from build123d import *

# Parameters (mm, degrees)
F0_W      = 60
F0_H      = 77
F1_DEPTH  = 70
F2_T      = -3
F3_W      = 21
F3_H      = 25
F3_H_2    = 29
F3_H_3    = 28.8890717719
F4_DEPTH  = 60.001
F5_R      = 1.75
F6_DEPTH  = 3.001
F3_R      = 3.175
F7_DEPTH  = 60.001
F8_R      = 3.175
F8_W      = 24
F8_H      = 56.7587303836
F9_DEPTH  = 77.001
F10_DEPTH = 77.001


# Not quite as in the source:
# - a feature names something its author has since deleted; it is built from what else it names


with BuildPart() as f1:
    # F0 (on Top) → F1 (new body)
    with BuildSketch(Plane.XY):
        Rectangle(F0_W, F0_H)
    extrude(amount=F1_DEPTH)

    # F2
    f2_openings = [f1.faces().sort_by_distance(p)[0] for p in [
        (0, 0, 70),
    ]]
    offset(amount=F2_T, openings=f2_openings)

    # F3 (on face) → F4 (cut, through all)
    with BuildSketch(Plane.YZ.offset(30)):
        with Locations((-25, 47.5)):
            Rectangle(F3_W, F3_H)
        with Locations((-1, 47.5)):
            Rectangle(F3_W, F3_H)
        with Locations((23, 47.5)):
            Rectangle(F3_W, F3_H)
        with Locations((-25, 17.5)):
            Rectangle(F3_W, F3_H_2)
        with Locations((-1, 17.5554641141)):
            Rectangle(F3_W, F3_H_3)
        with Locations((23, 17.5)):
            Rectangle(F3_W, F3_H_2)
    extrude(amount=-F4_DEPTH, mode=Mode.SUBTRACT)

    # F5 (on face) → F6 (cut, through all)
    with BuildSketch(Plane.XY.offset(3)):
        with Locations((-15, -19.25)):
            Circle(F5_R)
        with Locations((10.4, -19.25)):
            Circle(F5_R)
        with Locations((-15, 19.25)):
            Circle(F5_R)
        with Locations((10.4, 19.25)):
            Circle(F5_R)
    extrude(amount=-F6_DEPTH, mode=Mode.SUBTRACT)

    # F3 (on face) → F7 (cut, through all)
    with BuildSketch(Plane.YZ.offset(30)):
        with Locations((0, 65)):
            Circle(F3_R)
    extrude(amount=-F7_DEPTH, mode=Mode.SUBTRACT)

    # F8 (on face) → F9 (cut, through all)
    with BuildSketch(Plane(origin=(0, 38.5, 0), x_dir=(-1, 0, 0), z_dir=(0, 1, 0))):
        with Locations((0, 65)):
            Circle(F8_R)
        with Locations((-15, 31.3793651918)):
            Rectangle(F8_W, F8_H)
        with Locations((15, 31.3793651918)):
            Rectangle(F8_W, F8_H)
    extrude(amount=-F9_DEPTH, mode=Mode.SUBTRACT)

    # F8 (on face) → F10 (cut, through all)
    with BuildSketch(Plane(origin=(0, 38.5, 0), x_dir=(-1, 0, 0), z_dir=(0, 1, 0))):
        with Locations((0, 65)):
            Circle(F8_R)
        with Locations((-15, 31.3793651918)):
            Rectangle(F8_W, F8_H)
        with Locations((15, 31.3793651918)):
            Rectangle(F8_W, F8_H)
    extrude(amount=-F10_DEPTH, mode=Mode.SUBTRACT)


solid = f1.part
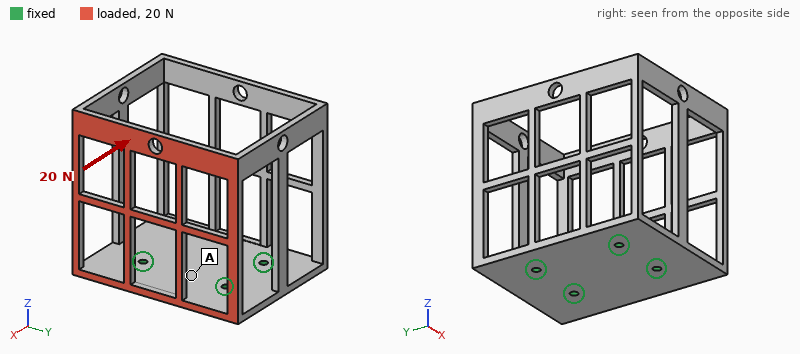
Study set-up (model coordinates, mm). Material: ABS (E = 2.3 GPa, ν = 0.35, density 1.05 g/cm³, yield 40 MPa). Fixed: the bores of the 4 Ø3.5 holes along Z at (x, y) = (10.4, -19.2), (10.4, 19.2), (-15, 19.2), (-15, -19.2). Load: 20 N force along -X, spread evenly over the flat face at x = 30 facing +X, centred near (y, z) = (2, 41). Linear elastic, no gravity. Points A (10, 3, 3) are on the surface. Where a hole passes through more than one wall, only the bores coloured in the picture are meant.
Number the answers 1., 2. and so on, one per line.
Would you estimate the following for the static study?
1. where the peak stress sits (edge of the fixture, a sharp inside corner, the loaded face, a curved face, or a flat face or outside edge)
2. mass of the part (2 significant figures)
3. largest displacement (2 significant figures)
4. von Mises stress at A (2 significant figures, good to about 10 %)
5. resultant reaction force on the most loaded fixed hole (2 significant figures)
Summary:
1. the loaded face
2. 31 g
3. 1.4 mm
4. 0.91 MPa
5. 13 N
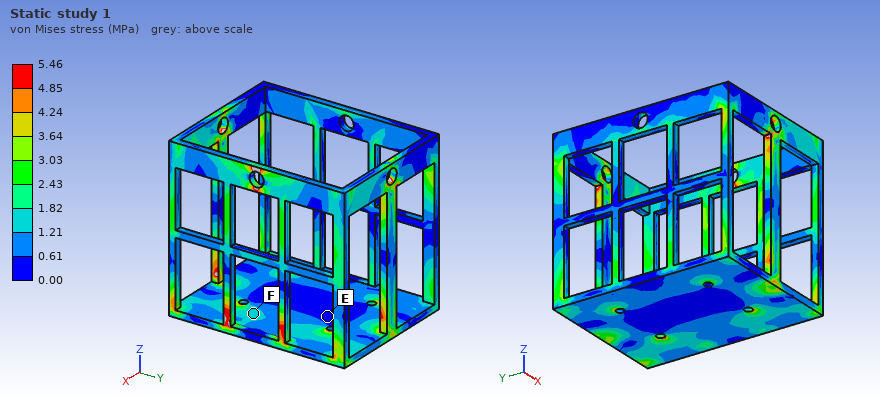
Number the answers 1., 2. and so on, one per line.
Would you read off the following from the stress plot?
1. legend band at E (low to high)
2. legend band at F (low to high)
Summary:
1. 0.00 to 0.61 MPa
2. 1.21 to 1.82 MPa
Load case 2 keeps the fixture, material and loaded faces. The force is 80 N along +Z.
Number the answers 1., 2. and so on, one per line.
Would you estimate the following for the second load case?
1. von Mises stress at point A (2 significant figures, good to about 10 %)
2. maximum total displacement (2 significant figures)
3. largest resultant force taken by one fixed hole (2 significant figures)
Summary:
1. 4.2 MPa
2. 0.96 mm
3. 57 N
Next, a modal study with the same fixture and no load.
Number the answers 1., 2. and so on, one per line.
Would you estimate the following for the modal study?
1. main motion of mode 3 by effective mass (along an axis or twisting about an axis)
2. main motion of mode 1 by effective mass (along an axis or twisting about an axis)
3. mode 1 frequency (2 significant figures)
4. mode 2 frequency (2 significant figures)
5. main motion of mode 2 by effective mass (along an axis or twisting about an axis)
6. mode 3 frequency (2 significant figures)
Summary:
1. twisting about Z
2. along X
3. 170 Hz
4. 210 Hz
5. along Y
6. 250 Hz
